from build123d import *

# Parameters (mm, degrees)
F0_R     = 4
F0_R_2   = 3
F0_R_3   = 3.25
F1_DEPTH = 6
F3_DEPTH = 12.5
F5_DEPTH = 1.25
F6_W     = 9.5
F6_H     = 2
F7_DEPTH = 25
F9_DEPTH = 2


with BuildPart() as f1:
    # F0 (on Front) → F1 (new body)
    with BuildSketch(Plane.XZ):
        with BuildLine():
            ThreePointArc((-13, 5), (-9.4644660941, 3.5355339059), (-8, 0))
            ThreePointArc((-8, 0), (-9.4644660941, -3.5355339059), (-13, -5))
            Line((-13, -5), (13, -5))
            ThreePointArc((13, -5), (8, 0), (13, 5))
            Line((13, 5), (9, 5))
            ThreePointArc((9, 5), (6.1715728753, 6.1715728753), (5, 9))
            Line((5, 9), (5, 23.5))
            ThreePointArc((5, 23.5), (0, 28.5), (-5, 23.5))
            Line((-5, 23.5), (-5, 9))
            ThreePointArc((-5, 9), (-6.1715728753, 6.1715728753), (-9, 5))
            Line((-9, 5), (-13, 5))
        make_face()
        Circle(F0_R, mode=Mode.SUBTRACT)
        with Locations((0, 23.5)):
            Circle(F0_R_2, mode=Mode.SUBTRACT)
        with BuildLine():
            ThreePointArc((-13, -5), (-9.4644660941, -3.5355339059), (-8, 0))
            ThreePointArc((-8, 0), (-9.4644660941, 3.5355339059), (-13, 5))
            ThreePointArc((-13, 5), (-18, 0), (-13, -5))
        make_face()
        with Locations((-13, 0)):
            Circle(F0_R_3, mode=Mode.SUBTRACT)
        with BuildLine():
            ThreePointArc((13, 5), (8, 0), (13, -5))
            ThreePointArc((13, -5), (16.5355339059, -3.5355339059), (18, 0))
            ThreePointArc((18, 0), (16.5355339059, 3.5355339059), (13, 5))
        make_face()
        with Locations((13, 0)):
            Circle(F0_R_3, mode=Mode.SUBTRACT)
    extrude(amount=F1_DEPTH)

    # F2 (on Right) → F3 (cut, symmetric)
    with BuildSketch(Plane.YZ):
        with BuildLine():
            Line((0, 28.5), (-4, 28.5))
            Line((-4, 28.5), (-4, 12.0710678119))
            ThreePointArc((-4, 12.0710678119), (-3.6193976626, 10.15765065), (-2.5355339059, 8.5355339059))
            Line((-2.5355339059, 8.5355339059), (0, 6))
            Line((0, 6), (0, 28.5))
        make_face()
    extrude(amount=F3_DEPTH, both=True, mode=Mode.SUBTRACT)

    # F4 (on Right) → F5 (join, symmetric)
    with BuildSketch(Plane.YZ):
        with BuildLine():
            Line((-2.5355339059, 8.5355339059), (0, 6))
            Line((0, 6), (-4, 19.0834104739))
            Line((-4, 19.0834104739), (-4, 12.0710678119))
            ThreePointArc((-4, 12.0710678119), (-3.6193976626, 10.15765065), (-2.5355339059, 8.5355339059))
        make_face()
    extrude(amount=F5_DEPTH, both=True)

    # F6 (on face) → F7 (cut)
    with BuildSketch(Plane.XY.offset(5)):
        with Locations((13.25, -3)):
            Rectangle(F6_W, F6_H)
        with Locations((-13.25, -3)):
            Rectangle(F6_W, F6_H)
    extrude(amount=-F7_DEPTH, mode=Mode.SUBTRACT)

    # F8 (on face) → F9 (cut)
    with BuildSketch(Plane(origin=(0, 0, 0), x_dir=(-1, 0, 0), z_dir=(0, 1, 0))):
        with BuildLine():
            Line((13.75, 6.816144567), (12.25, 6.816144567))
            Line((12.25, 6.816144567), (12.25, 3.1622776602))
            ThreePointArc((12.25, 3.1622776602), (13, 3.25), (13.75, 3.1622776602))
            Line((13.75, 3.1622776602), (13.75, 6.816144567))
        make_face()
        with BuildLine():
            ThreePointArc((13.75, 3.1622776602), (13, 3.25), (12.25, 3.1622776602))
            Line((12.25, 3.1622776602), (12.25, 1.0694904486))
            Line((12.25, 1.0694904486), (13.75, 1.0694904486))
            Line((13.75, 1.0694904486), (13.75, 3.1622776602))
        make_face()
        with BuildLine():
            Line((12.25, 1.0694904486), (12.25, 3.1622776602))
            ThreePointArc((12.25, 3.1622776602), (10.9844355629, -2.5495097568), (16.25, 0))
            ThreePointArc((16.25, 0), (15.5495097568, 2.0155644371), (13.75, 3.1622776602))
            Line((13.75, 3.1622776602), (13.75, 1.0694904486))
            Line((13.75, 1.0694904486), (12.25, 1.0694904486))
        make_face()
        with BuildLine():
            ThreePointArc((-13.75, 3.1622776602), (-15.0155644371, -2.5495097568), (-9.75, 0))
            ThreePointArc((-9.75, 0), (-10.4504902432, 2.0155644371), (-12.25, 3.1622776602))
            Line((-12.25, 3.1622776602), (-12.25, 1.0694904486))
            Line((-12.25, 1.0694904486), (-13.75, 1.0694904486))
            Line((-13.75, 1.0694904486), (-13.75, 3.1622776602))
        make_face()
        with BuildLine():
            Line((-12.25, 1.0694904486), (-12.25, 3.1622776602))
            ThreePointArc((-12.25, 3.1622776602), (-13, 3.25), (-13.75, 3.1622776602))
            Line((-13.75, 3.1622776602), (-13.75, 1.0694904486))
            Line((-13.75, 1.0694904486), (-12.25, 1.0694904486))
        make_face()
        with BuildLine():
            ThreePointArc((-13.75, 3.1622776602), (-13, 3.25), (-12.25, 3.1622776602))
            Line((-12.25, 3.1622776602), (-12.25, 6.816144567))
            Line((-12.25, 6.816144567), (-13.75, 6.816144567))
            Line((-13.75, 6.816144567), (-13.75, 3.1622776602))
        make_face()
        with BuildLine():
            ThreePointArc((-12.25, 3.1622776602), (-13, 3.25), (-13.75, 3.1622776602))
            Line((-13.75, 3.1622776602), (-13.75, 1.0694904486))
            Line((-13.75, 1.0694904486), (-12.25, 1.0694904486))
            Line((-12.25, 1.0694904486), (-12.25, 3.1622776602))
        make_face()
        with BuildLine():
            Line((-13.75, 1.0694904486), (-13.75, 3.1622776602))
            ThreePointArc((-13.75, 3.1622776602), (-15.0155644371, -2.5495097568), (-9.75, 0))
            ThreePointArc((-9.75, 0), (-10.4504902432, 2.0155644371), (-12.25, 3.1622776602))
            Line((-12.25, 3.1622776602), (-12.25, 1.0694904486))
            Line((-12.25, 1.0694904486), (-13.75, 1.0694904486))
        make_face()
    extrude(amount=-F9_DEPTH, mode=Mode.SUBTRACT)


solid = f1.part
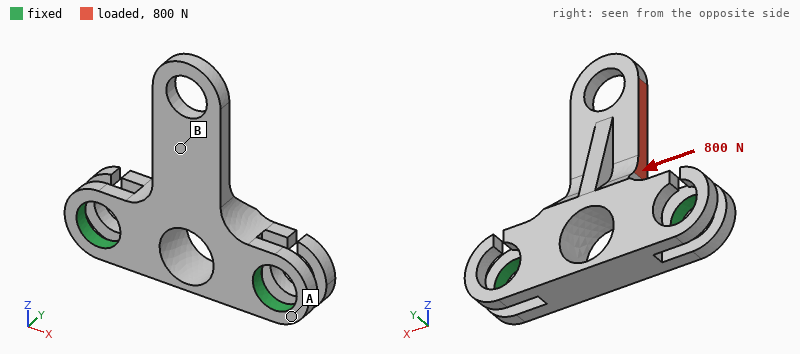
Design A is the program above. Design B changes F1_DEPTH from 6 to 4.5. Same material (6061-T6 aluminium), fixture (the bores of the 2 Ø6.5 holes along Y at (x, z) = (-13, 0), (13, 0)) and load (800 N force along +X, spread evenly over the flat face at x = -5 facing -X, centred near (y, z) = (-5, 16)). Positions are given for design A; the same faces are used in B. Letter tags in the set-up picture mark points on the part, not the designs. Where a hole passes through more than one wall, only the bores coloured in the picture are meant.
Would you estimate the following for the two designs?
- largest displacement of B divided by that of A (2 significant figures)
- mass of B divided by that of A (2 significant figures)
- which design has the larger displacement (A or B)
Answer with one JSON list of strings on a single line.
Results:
["2.5", "0.63", "B"]
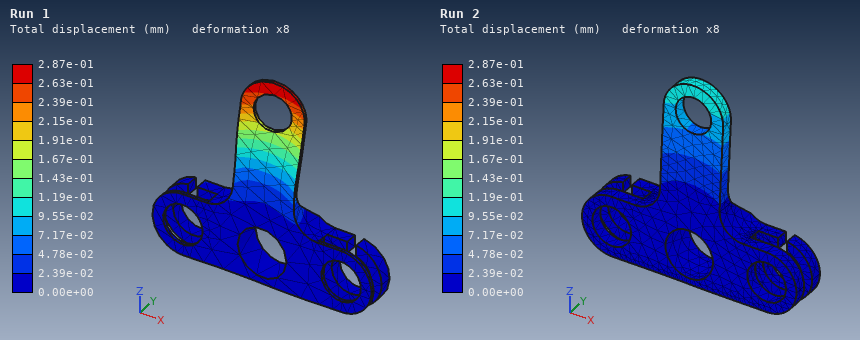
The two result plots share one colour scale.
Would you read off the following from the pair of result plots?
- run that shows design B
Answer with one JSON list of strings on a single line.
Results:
["Run 1"]
